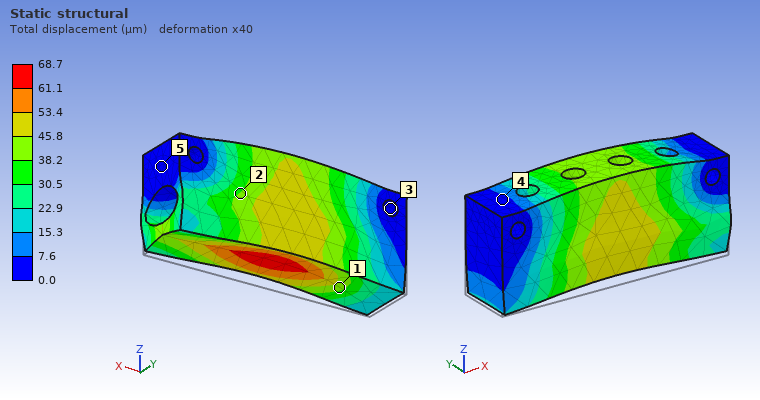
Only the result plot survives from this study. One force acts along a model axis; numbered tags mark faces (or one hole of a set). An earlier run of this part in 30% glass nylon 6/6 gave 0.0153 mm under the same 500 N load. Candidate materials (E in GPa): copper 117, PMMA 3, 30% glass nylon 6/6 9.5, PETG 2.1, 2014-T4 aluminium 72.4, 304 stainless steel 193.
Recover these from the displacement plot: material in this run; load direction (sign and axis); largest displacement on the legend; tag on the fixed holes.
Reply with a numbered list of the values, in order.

1. PETG
2. +Z
3. 68.7 µm
4. 3
